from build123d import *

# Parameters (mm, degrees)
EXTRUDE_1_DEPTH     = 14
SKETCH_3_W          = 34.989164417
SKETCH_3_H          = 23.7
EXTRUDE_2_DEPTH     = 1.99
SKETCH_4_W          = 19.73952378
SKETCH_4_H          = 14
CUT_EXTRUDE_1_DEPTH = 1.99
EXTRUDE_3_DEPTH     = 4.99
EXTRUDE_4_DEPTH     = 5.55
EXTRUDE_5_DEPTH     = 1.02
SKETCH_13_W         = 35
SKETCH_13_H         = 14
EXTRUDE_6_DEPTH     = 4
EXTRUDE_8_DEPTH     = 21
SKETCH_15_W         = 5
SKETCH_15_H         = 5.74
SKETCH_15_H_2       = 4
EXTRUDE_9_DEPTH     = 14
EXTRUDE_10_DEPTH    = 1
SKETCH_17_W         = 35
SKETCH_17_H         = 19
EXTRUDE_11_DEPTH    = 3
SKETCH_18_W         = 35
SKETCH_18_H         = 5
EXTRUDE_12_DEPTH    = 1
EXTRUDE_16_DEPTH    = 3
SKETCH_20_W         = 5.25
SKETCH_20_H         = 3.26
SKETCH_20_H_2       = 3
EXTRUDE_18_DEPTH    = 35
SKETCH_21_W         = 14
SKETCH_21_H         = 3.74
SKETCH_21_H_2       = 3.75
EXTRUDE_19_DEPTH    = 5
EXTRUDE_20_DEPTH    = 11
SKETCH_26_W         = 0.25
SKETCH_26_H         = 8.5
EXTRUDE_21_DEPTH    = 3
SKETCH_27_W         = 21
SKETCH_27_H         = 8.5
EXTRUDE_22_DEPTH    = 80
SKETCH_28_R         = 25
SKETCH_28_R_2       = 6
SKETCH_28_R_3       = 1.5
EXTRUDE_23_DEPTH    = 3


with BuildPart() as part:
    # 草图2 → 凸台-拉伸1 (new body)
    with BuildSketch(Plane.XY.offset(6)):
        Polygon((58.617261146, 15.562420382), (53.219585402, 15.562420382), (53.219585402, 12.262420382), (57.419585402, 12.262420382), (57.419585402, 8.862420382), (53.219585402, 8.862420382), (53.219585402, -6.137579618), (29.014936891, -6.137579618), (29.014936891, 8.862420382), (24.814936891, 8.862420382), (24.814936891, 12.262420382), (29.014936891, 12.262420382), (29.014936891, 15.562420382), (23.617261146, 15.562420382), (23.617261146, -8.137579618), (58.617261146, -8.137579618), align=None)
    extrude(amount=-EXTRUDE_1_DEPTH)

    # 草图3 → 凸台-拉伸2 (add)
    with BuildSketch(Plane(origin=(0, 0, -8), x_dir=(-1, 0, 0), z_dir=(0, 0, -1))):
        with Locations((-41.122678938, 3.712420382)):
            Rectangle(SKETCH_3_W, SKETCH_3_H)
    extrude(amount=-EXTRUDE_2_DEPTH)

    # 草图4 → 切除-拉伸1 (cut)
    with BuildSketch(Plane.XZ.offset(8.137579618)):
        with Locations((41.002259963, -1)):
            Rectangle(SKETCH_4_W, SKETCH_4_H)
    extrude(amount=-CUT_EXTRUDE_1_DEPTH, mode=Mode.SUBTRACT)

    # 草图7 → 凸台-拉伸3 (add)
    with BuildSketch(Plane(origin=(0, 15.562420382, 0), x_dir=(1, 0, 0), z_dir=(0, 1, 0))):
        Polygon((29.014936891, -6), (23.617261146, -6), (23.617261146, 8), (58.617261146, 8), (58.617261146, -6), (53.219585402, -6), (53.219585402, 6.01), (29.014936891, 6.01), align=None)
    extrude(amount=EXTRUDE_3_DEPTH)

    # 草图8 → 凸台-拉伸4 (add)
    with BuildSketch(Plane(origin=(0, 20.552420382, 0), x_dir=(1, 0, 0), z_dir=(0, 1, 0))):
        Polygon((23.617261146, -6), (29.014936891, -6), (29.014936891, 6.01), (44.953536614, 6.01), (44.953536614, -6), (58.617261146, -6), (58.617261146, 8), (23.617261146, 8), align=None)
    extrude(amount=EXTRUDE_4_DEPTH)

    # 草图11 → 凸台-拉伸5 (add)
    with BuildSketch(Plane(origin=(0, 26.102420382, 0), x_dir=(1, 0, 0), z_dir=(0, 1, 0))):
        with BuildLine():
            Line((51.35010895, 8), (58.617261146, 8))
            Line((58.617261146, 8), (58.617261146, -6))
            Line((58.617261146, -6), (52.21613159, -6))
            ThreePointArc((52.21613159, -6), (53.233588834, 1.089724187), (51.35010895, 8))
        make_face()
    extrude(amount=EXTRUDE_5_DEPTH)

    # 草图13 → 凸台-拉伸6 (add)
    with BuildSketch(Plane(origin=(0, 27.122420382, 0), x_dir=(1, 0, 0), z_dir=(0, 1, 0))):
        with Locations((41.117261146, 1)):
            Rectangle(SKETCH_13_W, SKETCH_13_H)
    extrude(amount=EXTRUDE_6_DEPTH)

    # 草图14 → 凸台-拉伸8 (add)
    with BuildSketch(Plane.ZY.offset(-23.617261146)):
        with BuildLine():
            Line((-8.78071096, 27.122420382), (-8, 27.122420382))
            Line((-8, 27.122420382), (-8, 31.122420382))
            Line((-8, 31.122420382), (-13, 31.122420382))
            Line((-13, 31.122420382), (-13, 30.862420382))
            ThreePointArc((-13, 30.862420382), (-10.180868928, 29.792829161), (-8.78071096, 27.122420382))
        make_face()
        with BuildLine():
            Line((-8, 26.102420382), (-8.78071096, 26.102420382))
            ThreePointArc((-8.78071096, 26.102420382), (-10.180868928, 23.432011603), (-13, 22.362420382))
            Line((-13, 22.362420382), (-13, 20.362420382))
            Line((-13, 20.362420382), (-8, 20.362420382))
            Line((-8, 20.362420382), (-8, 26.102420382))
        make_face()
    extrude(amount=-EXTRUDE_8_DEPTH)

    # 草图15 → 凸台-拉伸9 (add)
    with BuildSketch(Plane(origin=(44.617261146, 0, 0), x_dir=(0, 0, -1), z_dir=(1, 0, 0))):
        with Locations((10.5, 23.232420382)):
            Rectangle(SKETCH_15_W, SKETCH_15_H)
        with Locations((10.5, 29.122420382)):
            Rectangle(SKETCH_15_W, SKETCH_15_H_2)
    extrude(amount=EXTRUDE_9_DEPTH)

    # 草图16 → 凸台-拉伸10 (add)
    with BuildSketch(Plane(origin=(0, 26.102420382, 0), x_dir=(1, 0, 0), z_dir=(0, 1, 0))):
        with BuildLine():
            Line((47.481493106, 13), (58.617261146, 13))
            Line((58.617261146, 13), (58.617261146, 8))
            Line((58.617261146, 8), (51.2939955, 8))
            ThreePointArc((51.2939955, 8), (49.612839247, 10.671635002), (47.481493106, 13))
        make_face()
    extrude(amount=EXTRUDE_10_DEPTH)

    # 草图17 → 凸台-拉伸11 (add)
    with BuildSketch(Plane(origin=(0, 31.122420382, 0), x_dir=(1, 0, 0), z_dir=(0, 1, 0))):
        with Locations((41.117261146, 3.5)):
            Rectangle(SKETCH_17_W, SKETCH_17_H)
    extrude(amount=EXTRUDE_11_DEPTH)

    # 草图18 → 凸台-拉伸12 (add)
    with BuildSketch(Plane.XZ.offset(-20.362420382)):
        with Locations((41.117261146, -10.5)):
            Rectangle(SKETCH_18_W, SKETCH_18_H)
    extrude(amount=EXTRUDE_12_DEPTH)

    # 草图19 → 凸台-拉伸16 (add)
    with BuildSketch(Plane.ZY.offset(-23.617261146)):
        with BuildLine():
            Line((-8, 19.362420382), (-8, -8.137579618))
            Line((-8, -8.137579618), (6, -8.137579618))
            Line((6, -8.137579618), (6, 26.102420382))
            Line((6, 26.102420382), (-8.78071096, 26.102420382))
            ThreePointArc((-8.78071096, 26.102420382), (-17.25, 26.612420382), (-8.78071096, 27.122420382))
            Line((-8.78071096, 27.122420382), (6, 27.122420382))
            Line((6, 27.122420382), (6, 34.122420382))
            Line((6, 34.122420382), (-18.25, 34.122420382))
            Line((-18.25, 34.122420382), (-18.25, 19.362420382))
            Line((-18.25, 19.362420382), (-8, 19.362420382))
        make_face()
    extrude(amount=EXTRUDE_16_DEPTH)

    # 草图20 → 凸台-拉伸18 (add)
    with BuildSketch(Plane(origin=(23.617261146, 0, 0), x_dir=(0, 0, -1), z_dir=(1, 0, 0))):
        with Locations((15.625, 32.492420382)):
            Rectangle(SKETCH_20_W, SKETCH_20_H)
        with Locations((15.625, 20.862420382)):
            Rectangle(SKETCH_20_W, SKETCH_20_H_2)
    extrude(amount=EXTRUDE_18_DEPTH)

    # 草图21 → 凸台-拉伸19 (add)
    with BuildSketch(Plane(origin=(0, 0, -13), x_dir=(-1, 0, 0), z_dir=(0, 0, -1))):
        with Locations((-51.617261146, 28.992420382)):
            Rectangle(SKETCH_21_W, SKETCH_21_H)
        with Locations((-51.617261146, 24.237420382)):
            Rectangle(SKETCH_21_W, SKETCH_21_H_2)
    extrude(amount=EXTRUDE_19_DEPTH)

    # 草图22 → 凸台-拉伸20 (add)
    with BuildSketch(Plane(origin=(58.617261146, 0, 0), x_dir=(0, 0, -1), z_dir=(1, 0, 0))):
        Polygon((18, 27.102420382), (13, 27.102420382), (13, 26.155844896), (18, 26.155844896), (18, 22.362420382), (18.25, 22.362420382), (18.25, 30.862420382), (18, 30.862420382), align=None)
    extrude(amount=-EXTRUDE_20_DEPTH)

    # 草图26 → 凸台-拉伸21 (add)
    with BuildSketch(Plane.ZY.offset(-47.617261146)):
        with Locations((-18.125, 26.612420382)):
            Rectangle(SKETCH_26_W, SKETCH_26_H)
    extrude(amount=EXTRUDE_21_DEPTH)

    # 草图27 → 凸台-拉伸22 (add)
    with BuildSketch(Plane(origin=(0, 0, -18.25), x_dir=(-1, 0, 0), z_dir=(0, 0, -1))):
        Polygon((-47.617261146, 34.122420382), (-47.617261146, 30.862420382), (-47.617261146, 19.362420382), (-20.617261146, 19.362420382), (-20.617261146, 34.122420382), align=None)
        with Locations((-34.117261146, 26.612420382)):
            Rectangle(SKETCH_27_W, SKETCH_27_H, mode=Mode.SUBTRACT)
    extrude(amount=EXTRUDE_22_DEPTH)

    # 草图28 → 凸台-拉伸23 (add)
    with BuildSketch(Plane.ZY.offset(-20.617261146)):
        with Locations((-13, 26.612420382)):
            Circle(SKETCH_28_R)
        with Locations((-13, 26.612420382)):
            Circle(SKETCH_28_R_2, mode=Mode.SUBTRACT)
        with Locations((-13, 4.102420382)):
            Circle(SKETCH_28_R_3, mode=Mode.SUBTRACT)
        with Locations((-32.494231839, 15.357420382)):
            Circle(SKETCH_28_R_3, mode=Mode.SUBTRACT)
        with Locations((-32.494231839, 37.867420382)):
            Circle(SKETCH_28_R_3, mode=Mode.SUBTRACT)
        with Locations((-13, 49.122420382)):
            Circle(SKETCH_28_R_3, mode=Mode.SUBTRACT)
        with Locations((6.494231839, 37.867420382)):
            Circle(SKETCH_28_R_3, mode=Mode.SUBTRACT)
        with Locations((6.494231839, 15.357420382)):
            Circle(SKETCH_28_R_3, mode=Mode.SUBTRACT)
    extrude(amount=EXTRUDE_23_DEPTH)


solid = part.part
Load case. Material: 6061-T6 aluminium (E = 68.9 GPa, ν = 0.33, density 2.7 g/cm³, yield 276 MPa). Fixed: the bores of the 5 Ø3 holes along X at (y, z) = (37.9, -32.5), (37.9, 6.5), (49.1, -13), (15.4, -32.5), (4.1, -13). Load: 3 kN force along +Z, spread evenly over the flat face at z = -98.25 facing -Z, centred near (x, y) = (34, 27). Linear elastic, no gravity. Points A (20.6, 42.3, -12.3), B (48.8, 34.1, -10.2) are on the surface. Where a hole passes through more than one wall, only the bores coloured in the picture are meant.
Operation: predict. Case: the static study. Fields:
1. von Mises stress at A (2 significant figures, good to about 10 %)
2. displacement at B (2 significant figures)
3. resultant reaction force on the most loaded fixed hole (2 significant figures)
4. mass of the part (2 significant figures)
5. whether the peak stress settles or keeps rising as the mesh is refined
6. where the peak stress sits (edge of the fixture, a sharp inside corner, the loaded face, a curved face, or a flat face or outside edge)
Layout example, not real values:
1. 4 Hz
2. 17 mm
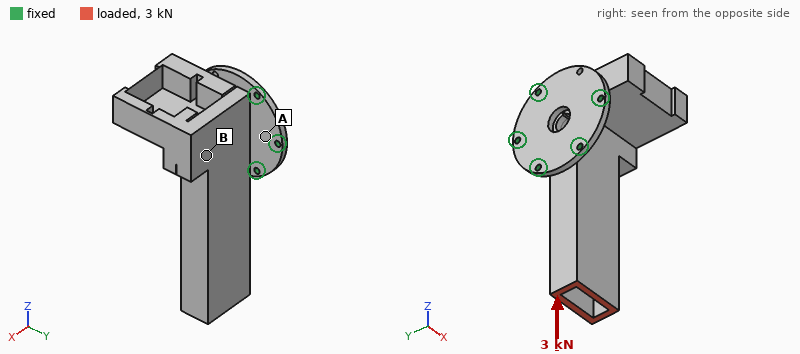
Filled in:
1. 16 MPa
2. 0.038 mm
3. 1.2 kN
4. 110 g
5. keeps rising
6. edge of the fixture
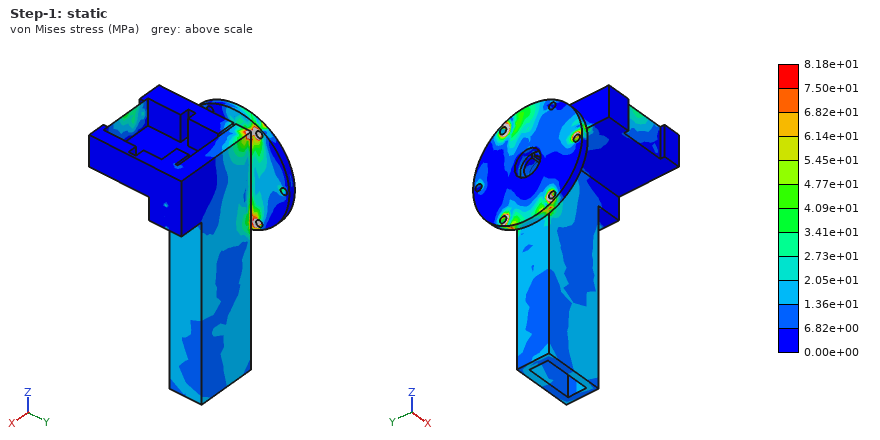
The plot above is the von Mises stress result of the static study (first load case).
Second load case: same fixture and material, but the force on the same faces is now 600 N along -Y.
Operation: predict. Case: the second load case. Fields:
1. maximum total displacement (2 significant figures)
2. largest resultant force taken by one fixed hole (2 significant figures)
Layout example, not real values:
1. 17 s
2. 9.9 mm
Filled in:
1. 0.29 mm
2. 1.1 kN
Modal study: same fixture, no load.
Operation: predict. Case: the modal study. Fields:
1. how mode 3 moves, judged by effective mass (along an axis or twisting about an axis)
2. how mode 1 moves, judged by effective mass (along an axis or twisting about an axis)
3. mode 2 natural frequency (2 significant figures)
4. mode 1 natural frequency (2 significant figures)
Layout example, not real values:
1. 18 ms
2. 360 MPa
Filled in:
1. along Y
2. along Y
3. 2400 Hz
4. 2000 Hz
